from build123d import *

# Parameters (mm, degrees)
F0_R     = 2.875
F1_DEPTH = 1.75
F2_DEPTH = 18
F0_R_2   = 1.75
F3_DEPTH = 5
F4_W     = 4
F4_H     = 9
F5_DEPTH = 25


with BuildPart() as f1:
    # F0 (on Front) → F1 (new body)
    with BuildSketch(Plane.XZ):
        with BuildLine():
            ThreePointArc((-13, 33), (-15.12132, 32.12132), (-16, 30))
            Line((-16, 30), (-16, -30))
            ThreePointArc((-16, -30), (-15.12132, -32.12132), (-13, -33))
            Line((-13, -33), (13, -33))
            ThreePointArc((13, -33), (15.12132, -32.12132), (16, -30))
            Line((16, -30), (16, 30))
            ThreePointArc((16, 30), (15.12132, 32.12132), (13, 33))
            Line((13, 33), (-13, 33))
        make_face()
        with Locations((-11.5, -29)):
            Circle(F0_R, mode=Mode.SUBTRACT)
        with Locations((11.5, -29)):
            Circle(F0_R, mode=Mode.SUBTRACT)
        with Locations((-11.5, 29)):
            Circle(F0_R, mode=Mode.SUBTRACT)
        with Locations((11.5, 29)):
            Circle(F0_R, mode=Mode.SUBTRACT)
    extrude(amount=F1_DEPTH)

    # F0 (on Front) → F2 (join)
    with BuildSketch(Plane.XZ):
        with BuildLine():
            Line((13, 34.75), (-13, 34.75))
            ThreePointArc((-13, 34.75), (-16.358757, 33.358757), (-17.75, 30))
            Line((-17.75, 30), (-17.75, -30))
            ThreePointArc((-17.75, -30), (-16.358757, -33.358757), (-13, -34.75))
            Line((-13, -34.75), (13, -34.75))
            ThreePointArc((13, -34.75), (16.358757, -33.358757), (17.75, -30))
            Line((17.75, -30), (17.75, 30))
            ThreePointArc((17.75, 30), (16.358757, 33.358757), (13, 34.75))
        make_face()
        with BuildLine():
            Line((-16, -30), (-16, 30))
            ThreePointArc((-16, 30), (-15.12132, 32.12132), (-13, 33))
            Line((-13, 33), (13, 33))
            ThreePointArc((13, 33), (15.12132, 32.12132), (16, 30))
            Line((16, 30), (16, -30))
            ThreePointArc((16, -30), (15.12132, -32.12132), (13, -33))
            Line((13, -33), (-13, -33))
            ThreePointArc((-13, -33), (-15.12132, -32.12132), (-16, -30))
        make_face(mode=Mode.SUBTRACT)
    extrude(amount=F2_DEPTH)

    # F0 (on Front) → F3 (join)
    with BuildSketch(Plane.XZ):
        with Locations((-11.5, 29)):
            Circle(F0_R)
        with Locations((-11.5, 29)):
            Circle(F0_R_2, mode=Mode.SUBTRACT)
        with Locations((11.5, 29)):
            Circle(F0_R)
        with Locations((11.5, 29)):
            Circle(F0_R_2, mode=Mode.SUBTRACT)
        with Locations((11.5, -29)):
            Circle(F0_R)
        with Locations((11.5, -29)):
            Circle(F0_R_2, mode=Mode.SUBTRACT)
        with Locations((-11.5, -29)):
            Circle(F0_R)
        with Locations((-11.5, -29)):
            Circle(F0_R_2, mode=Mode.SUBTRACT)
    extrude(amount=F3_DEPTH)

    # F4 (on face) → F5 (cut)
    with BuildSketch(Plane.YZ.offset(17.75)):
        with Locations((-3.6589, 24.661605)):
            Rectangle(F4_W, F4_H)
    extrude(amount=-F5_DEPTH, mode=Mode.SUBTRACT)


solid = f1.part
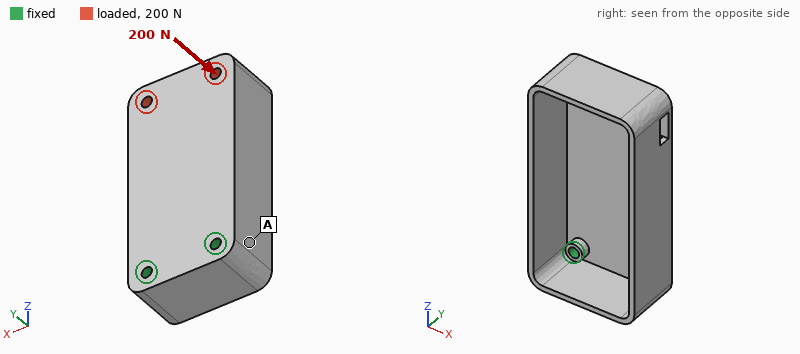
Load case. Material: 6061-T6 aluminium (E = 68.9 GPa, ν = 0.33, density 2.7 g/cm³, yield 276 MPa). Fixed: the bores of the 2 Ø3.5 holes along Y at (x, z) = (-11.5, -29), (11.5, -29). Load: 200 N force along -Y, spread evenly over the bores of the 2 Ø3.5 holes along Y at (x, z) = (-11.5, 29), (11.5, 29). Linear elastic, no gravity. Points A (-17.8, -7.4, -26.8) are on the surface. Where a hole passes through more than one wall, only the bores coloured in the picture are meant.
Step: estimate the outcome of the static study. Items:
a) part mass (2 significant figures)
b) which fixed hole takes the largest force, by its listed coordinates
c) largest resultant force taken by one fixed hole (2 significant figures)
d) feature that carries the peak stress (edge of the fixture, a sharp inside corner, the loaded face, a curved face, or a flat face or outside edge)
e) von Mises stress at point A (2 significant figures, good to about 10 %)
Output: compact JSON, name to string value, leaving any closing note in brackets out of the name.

{"part mass": "27 g", "which fixed hole takes the largest force, by its listed coordinates": "(-11.5, -29)", "largest resultant force taken by one fixed hole": "150 N", "feature that carries the peak stress": "a flat face or outside edge", "von Mises stress at point A": "31 MPa"}
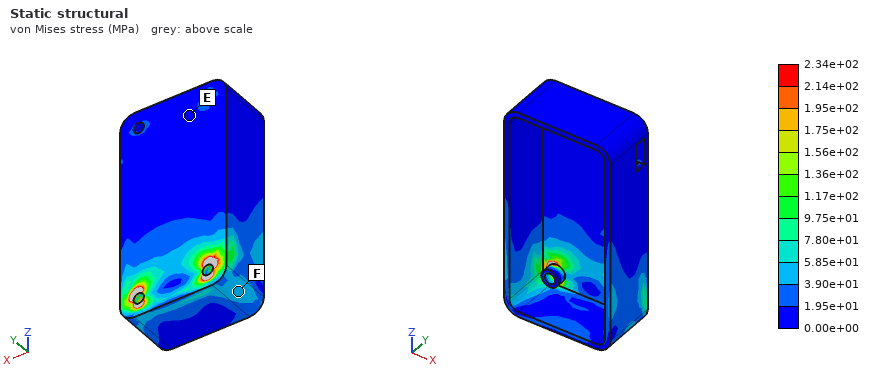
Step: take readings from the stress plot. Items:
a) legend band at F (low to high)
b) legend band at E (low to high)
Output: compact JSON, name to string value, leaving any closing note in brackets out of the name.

{"legend band at F": "3.90e+01 to 5.85e+01 MPa", "legend band at E": "0.00e+00 to 1.95e+01 MPa"}
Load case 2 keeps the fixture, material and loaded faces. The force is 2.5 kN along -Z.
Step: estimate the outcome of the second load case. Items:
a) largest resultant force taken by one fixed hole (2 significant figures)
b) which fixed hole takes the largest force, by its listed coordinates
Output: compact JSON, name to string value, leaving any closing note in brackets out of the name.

{"largest resultant force taken by one fixed hole": "1.5 kN", "which fixed hole takes the largest force, by its listed coordinates": "(-11.5, -29)"}
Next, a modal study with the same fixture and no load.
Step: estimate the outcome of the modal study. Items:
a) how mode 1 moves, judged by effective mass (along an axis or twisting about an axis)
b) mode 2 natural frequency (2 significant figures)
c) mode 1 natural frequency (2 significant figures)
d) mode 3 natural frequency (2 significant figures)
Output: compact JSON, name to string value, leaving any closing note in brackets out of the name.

{"how mode 1 moves, judged by effective mass": "along Y", "mode 2 natural frequency": "1200 Hz", "mode 1 natural frequency": "800 Hz", "mode 3 natural frequency": "3800 Hz"}
